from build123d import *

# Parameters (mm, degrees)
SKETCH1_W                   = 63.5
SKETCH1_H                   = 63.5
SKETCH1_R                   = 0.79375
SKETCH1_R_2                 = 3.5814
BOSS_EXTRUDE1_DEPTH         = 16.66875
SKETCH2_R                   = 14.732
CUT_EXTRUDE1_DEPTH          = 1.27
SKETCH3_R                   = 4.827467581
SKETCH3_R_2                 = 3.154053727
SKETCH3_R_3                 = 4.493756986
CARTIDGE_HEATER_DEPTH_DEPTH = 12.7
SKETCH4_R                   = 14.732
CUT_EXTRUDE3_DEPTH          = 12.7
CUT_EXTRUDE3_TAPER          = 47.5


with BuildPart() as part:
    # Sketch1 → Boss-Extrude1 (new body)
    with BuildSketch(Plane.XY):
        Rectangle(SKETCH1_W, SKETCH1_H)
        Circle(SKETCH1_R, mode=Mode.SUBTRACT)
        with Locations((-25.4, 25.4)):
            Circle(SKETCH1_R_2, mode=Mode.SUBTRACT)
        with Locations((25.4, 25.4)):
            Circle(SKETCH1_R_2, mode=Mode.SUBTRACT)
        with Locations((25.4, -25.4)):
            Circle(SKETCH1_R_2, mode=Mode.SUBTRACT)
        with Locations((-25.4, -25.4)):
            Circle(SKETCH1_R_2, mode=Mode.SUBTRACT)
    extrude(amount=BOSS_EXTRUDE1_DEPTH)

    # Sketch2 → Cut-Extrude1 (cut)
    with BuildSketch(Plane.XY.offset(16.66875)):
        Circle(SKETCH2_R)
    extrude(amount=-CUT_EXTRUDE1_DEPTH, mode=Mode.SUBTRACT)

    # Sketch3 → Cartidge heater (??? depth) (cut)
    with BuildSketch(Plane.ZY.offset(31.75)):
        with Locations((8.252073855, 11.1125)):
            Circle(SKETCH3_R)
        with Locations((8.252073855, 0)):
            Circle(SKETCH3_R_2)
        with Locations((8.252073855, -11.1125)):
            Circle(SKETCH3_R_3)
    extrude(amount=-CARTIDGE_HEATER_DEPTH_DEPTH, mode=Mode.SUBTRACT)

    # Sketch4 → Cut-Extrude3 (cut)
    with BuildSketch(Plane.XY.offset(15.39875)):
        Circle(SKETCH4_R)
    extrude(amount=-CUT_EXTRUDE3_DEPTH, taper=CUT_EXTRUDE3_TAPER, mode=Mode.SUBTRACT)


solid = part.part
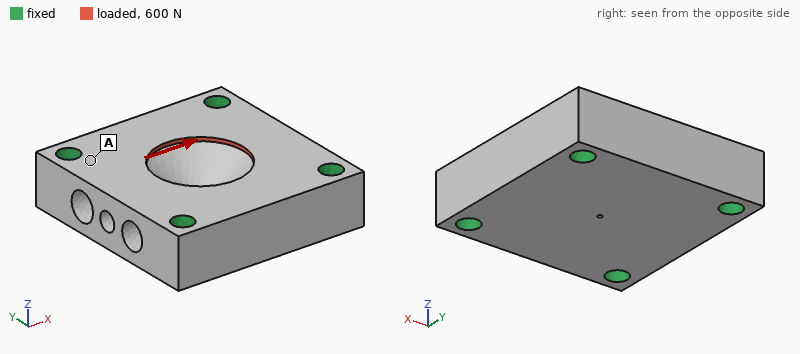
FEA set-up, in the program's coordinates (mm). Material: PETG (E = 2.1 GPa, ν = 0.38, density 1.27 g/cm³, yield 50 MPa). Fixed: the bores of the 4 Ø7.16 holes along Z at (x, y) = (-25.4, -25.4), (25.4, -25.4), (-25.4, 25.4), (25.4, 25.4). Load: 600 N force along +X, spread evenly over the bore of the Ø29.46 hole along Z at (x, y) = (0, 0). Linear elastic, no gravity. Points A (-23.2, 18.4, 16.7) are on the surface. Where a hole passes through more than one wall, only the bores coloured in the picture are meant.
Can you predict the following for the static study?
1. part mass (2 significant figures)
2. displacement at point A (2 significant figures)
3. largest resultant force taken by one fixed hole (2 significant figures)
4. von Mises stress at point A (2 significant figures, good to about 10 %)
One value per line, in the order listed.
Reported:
74 g
3.5 µm
170 N
0.84 MPa
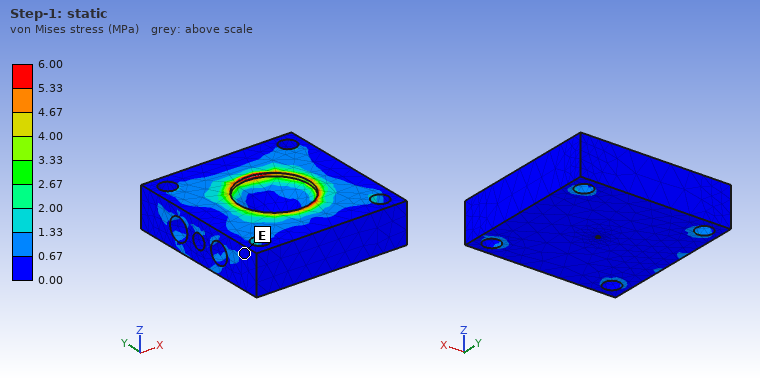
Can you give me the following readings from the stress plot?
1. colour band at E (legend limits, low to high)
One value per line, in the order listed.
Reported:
0.00 to 0.67 MPa
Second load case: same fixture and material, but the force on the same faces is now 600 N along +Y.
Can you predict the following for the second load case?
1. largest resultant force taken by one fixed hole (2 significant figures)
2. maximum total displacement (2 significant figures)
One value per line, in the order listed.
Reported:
180 N
20 µm
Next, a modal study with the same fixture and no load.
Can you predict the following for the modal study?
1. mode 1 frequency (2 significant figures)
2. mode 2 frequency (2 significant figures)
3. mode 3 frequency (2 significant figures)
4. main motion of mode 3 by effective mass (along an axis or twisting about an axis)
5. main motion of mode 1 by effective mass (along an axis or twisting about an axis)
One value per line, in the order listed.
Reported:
4200 Hz
5600 Hz
6100 Hz
twisting about X
along Z
